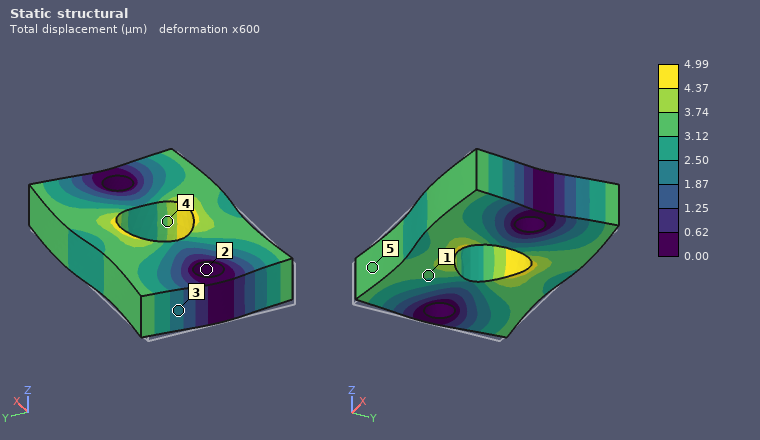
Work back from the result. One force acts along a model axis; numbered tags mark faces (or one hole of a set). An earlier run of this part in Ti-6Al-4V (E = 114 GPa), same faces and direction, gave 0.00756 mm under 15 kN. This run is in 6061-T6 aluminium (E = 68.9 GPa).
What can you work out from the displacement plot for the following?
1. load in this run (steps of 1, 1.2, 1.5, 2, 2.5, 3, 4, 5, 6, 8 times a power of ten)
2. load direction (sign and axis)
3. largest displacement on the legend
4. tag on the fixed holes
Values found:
6 kN
+X
4.99 µm
2
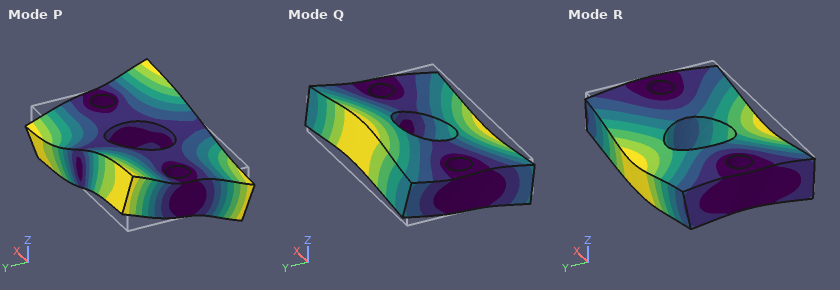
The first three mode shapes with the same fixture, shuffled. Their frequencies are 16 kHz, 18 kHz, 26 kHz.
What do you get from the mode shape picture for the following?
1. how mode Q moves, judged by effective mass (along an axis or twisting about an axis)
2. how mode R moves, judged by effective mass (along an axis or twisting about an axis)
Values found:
twisting about X
along Z
